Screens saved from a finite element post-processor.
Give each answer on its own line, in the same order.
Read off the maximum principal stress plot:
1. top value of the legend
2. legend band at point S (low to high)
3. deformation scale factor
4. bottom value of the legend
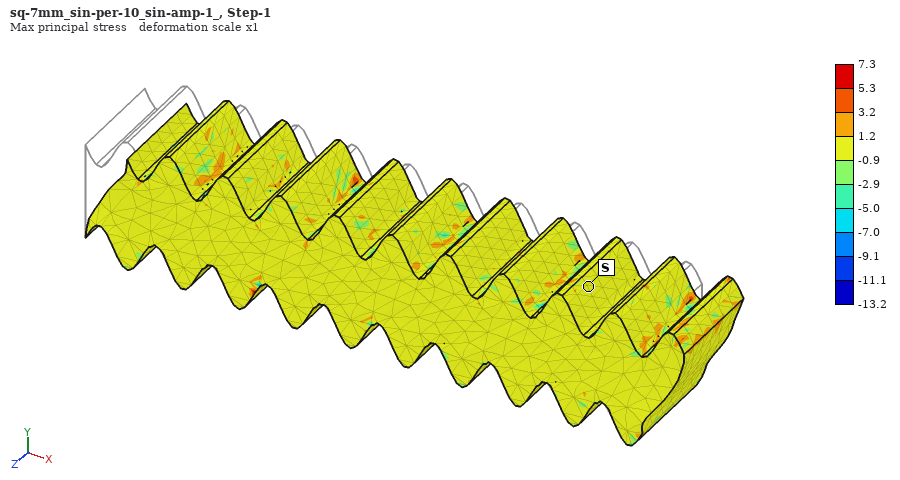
7.3
-0.9 to 1.2
1
-13.2
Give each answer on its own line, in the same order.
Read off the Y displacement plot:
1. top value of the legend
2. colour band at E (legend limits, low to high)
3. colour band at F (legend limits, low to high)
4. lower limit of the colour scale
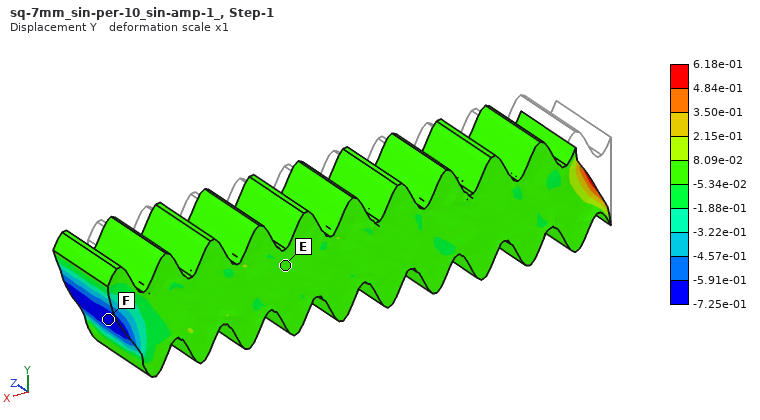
6.18e-01
-5.34e-02 to 8.09e-02
-7.25e-01 to -5.91e-01
-7.25e-01
